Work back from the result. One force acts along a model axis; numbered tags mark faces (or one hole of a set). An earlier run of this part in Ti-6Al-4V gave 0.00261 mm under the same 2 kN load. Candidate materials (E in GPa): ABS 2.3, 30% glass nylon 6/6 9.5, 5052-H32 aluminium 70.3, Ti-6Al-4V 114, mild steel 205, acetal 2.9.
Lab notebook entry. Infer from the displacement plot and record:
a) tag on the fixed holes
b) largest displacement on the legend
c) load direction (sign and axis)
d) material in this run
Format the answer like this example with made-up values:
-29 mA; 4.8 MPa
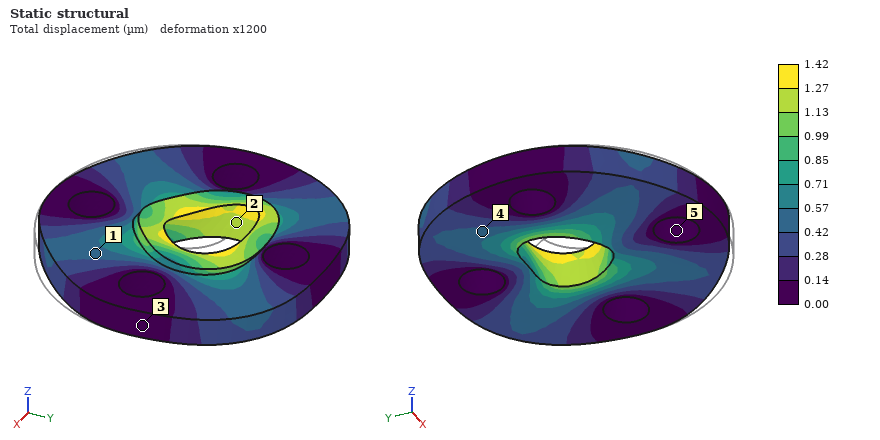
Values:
5; 1.42 µm; +Y; mild steel
